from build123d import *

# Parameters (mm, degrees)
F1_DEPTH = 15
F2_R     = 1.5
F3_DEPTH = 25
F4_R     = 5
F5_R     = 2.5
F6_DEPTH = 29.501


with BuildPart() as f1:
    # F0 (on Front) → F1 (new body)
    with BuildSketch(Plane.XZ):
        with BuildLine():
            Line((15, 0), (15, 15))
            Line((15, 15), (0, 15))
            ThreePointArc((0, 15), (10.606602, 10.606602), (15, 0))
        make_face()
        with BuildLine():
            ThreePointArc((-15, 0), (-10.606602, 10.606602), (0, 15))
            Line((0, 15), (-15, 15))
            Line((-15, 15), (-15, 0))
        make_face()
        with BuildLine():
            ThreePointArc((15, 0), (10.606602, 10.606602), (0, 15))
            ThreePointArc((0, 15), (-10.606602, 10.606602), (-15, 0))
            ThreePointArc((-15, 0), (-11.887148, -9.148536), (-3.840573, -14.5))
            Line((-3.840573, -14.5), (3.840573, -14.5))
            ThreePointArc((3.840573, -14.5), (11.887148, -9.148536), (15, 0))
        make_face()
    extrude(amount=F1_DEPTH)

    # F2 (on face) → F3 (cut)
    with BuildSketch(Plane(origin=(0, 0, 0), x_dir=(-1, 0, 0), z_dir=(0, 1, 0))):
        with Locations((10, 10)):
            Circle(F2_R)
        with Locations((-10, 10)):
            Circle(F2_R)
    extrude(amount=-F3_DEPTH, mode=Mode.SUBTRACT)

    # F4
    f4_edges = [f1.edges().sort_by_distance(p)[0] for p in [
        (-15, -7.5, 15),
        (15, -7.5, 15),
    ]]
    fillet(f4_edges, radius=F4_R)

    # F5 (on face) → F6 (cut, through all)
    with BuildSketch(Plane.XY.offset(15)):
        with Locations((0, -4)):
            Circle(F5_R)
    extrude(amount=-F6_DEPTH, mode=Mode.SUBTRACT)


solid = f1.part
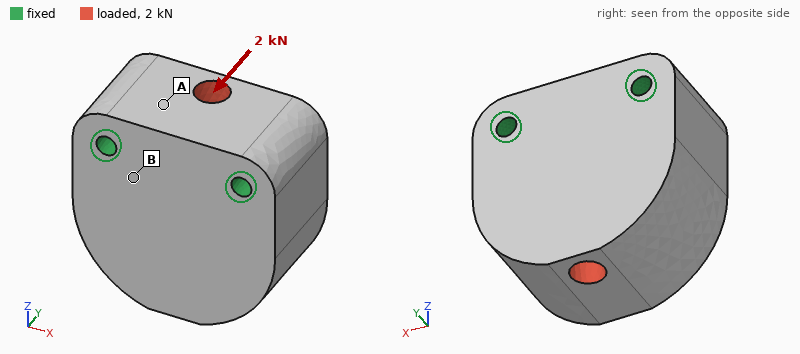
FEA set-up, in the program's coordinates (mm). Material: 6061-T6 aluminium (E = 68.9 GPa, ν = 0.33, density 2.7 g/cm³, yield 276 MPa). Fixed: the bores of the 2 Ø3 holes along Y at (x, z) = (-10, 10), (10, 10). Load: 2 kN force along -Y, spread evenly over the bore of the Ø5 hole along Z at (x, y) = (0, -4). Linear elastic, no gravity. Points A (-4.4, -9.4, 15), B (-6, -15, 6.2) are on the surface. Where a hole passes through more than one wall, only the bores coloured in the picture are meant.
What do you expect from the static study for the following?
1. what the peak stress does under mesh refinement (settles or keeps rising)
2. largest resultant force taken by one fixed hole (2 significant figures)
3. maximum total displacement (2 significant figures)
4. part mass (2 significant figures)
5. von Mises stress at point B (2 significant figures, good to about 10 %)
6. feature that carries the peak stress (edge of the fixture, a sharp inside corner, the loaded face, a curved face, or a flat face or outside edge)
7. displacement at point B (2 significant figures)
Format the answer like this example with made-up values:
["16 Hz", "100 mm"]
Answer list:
["keeps rising", "1.0 kN", "13 µm", "30 g", "12 MPa", "edge of the fixture", "2.6 µm"]
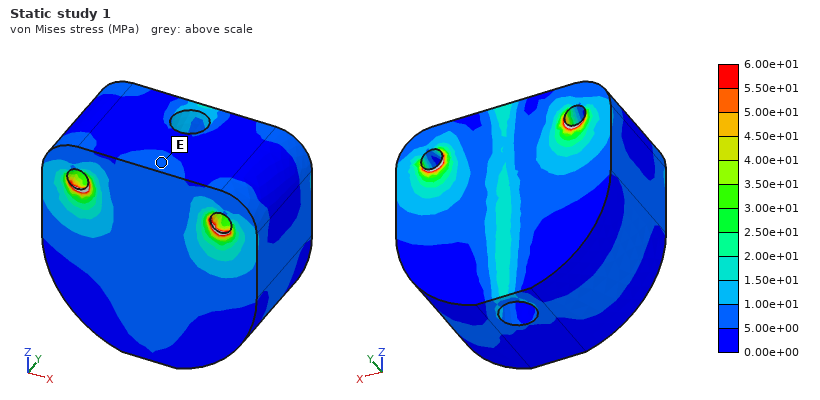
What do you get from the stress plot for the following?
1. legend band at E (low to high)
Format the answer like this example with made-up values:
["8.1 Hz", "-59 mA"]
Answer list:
["5.00e+00 to 1.00e+01 MPa"]
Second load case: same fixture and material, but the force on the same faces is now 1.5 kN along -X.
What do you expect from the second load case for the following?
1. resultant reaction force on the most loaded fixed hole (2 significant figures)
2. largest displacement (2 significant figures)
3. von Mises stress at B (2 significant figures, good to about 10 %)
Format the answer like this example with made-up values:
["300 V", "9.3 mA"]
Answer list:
["1.0 kN", "4.0 µm", "3.9 MPa"]
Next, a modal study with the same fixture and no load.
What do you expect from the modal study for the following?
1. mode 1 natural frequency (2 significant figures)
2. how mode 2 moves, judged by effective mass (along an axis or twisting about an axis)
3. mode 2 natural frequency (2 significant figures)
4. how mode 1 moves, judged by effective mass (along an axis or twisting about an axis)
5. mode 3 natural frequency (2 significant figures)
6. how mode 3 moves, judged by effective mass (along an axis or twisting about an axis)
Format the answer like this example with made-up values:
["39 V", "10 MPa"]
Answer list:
["17 kHz", "along X", "25 kHz", "along Y", "32 kHz", "twisting about Z"]
